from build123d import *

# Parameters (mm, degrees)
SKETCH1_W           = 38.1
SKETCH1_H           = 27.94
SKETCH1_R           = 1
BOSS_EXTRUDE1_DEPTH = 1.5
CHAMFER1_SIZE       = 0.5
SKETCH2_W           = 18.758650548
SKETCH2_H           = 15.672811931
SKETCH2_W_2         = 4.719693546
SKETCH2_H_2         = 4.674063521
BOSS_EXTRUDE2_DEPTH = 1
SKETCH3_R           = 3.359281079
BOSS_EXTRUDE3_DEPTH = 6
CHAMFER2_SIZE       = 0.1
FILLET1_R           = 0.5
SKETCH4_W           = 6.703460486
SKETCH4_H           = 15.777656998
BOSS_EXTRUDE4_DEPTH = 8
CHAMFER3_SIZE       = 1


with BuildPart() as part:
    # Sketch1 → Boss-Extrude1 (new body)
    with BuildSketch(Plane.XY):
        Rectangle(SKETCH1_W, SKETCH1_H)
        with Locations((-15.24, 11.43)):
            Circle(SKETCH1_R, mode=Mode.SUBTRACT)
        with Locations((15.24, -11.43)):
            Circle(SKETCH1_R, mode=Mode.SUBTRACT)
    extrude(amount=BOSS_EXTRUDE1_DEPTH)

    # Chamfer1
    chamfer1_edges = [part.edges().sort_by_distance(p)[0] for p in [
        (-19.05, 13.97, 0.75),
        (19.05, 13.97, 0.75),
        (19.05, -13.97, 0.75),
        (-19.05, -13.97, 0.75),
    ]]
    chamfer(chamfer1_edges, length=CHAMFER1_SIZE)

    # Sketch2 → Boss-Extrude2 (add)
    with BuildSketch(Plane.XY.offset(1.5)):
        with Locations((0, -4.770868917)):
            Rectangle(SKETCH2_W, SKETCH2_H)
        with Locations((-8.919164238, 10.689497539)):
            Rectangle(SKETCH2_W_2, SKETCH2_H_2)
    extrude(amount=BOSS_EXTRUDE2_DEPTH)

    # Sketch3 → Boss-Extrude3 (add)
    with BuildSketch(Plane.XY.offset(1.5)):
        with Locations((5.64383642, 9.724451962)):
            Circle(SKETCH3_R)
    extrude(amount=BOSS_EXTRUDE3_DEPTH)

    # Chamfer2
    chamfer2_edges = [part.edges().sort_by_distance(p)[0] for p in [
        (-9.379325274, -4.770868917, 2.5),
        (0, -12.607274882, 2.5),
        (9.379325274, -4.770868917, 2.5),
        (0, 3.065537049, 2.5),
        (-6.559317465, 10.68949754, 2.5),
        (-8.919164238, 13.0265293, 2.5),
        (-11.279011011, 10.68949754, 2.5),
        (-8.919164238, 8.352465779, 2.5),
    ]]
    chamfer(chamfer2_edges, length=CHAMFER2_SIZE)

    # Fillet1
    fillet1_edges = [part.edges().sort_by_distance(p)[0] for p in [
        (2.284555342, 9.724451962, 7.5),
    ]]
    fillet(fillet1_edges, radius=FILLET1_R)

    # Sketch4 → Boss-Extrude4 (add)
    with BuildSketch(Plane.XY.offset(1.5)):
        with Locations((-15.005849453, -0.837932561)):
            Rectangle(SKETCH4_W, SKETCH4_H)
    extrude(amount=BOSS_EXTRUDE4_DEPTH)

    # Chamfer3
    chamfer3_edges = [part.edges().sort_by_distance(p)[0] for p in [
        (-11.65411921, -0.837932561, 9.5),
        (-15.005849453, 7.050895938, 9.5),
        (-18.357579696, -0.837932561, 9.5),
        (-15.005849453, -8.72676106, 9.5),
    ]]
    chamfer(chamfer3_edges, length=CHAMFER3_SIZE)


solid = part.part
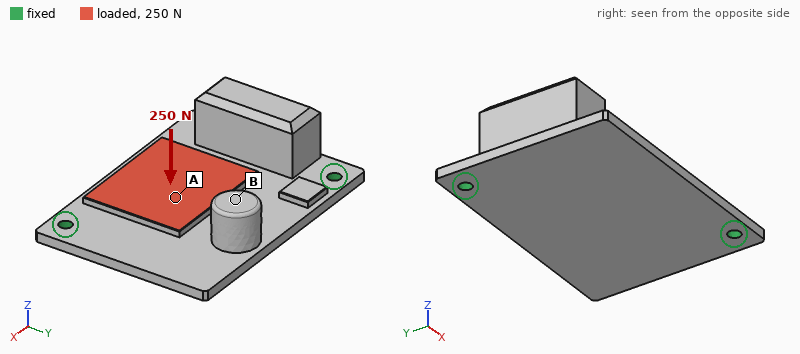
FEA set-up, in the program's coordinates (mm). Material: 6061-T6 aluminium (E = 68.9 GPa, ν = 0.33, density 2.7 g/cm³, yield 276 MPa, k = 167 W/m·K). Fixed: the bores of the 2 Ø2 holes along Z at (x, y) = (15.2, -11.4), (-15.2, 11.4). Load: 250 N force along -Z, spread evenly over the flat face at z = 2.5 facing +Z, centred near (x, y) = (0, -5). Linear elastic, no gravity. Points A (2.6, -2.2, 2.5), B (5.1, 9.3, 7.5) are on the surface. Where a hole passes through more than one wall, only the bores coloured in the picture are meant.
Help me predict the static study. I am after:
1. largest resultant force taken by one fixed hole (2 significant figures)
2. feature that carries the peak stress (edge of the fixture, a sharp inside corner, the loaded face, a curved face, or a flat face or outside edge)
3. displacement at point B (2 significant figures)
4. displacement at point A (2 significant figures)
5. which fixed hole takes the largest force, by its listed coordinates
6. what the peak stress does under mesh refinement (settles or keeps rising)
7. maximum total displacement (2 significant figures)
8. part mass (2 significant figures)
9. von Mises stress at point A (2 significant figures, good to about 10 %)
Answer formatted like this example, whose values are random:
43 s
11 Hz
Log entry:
210 N
edge of the fixture
0.048 mm
0.084 mm
(15.2, -11.4)
keeps rising
0.26 mm
7.9 g
58 MPa
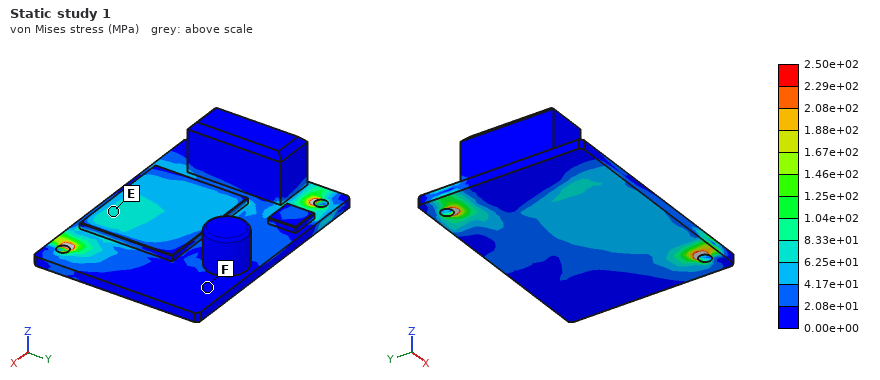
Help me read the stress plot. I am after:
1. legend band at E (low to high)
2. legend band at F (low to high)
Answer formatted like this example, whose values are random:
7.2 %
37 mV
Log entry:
6.25e+01 to 8.33e+01 MPa
0.00e+00 to 2.08e+01 MPa
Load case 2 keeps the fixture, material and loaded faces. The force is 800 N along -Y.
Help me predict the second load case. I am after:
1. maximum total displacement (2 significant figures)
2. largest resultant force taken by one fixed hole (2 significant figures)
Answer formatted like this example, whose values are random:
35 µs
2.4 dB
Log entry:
0.23 mm
400 N
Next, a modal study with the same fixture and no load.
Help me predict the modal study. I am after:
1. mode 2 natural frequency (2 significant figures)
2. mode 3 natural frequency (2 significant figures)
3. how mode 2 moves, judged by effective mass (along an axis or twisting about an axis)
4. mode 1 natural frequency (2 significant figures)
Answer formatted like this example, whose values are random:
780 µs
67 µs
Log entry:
3200 Hz
6600 Hz
along Z
1900 Hz
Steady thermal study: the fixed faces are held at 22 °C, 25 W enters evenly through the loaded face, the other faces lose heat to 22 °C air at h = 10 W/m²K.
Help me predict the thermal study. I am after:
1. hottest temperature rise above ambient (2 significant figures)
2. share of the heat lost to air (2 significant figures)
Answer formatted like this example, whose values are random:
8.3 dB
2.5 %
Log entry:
44 K
3.1 %
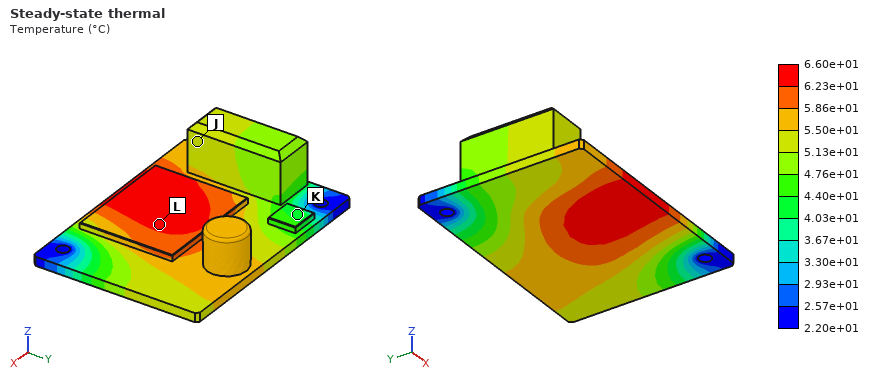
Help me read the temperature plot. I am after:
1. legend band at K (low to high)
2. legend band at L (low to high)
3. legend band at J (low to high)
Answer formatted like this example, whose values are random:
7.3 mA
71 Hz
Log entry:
4.03e+01 to 4.40e+01 °C
6.23e+01 to 6.60e+01 °C
5.13e+01 to 5.50e+01 °C
